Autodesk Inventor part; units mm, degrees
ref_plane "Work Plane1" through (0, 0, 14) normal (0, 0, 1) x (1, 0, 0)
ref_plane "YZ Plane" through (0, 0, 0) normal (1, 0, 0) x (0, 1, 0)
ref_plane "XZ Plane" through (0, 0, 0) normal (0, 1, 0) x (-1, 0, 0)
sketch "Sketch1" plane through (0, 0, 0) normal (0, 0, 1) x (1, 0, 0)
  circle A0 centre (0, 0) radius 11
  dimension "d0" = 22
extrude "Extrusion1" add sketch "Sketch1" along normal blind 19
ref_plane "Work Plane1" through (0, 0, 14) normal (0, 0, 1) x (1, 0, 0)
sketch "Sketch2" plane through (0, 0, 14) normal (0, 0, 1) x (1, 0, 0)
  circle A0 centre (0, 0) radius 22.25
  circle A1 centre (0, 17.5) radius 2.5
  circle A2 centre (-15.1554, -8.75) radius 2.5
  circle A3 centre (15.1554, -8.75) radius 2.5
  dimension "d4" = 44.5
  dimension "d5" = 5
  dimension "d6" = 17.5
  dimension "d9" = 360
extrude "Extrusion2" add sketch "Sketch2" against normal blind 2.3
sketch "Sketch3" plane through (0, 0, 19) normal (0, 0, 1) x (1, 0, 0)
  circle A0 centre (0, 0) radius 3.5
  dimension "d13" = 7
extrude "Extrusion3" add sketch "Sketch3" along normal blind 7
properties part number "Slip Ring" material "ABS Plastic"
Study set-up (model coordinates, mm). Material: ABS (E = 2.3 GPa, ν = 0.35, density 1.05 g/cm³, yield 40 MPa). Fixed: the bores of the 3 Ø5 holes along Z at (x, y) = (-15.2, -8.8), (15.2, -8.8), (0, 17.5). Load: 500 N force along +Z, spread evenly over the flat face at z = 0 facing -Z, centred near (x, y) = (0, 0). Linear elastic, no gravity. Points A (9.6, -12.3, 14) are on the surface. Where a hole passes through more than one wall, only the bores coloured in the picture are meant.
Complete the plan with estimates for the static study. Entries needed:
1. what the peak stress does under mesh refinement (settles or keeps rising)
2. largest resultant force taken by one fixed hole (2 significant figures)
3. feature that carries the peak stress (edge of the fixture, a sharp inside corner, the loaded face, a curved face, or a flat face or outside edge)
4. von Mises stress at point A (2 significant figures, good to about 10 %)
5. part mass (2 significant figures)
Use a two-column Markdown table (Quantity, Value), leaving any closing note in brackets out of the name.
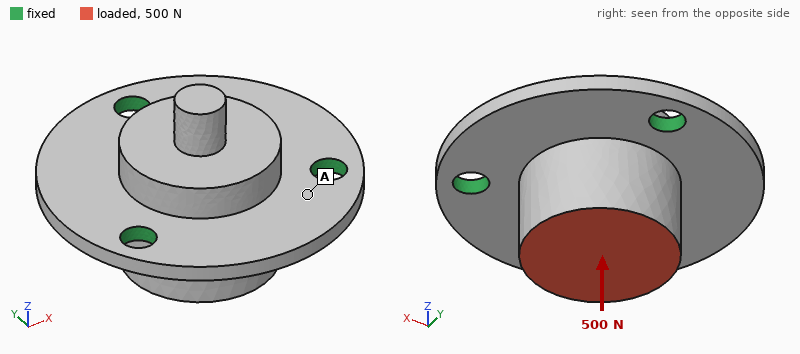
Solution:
| Quantity | Value |
|---|---|
| what the peak stress does under mesh refinement | keeps rising |
| largest resultant force taken by one fixed hole | 170 N |
| feature that carries the peak stress | edge of the fixture |
| von Mises stress at point A | 5.2 MPa |
| part mass | 11 g |
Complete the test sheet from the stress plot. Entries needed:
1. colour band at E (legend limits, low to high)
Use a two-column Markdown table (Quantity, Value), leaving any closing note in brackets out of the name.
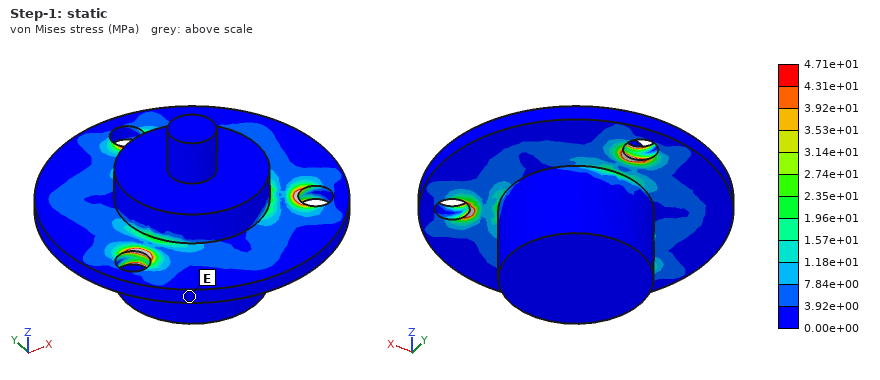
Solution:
| Quantity | Value |
|---|---|
| colour band at E | 0.00e+00 to 3.92e+00 MPa |
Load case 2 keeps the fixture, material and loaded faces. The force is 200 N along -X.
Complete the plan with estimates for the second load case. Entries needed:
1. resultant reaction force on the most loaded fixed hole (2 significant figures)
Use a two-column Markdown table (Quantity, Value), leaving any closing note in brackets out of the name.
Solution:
| Quantity | Value |
|---|---|
| resultant reaction force on the most loaded fixed hole | 130 N |
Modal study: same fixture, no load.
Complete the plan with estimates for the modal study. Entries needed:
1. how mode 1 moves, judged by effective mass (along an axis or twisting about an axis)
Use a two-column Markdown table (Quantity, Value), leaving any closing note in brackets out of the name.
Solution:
| Quantity | Value |
|---|---|
| how mode 1 moves, judged by effective mass | along Z |
